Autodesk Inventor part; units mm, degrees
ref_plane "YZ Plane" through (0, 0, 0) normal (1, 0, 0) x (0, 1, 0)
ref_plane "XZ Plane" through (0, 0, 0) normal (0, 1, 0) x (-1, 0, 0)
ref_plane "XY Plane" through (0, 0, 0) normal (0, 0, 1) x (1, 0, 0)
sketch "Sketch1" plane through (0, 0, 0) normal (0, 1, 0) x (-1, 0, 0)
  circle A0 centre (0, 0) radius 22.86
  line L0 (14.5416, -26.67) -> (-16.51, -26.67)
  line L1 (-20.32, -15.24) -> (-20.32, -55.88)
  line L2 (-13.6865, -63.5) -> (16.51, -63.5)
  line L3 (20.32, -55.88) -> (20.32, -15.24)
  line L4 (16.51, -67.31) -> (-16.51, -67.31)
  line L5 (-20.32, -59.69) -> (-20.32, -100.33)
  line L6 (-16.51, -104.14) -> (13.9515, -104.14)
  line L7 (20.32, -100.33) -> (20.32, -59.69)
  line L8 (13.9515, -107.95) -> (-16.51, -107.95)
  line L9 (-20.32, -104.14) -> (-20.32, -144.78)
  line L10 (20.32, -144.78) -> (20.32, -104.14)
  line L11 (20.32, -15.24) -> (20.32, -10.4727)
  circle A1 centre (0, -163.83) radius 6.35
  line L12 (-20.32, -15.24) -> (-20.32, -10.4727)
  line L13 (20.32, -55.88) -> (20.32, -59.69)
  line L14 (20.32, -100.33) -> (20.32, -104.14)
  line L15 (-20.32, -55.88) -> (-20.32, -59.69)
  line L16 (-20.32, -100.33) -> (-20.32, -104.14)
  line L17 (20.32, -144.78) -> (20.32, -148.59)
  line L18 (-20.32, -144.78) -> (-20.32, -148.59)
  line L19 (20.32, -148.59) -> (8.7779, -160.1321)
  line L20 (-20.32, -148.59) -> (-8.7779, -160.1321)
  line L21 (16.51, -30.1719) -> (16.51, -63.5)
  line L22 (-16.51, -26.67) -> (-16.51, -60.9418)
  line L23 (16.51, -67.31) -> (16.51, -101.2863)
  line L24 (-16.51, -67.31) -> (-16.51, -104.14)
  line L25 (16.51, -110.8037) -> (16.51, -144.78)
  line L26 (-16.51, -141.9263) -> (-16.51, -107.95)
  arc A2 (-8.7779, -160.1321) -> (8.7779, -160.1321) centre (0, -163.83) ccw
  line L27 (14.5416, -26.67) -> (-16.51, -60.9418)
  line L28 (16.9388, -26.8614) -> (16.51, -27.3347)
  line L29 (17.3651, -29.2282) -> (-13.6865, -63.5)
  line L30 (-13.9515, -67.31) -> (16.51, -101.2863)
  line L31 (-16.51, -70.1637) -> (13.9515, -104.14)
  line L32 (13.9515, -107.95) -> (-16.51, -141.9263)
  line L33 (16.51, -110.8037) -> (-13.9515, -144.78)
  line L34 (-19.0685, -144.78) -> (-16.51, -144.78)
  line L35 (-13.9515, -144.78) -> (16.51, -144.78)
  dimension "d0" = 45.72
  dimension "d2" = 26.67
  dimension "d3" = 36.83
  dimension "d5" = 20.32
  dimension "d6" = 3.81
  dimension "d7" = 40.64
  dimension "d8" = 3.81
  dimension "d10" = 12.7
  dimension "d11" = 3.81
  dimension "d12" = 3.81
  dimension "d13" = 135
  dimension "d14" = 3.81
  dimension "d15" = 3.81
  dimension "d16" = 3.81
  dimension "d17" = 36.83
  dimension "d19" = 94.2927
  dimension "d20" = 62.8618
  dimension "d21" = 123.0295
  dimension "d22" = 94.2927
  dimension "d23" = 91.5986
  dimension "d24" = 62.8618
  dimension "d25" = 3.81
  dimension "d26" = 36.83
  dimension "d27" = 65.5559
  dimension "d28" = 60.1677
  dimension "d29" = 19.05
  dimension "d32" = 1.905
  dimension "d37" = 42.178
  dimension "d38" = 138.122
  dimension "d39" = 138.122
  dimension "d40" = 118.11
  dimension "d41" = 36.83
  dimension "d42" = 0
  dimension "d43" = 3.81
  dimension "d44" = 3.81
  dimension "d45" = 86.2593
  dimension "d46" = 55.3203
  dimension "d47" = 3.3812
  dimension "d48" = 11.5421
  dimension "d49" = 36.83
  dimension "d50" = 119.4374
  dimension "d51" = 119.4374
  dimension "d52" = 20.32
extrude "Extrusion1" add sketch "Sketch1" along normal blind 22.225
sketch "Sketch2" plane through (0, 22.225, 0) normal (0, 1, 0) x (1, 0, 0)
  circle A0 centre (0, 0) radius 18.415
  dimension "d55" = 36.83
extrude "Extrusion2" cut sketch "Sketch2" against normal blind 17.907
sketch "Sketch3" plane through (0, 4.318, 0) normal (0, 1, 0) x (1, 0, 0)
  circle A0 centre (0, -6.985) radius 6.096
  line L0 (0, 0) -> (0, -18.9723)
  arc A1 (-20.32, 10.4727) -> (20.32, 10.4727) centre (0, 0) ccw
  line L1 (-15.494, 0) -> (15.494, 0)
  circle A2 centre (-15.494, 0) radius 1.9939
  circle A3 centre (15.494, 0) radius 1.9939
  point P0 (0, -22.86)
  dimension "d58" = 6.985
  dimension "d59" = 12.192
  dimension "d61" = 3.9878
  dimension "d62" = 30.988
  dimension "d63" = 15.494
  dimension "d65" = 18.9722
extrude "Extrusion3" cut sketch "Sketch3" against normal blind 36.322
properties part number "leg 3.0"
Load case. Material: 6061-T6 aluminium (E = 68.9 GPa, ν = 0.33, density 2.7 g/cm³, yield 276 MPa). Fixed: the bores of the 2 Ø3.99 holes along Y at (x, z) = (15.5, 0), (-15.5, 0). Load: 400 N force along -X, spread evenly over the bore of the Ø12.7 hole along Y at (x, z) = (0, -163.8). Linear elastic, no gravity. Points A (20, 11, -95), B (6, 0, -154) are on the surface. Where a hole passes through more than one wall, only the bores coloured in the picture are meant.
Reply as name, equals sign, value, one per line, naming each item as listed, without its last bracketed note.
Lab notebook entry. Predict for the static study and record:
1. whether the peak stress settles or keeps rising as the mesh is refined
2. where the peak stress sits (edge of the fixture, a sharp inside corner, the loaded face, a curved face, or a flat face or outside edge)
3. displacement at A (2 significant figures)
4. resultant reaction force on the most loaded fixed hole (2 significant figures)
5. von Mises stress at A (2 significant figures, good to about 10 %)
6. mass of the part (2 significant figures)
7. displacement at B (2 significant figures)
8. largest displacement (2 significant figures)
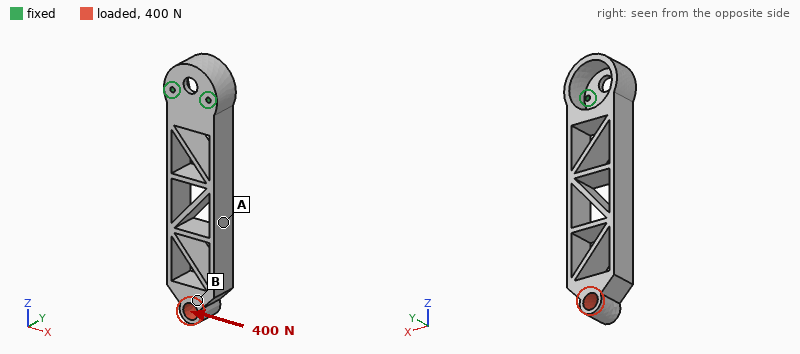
whether the peak stress settles or keeps rising as the mesh is refined = keeps rising
where the peak stress sits = edge of the fixture
displacement at A = 0.10 mm
resultant reaction force on the most loaded fixed hole = 2.0 kN
von Mises stress at A = 7.6 MPa
mass of the part = 200 g
displacement at B = 0.20 mm
largest displacement = 0.24 mm
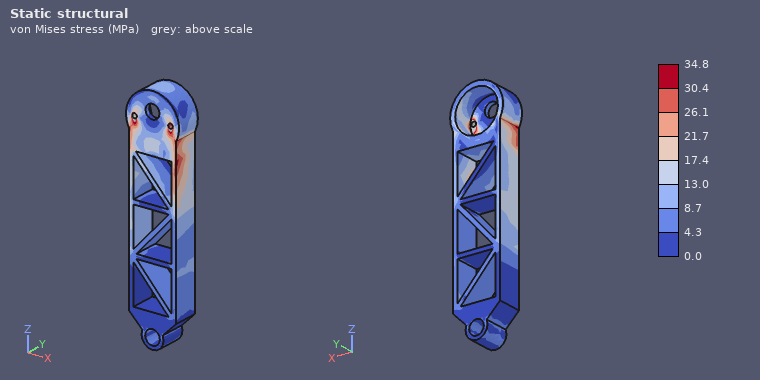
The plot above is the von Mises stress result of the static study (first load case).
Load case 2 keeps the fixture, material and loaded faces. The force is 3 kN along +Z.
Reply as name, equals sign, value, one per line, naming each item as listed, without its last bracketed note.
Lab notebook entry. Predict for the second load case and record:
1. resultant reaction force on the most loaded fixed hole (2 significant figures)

resultant reaction force on the most loaded fixed hole = 1.5 kN
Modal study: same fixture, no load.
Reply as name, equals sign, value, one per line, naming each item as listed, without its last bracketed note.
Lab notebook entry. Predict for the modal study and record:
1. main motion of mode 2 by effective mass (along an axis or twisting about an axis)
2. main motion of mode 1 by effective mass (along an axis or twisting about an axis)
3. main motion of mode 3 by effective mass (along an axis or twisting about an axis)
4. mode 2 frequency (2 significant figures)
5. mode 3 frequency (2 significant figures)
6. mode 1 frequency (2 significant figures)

main motion of mode 2 by effective mass = along X
main motion of mode 1 by effective mass = along Y
main motion of mode 3 by effective mass = twisting about Z
mode 2 frequency = 940 Hz
mode 3 frequency = 2000 Hz
mode 1 frequency = 280 Hz
